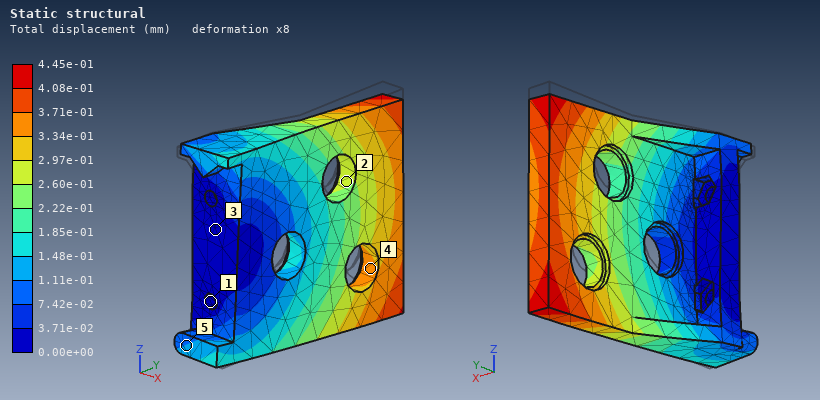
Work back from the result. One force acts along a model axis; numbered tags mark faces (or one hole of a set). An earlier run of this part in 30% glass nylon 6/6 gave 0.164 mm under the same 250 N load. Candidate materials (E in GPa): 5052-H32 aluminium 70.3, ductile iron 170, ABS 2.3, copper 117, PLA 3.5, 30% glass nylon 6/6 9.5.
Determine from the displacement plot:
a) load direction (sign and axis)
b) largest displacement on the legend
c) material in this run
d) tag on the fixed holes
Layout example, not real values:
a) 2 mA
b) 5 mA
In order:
a) -Z
b) 4.45e-01 mm
c) PLA
d) 1
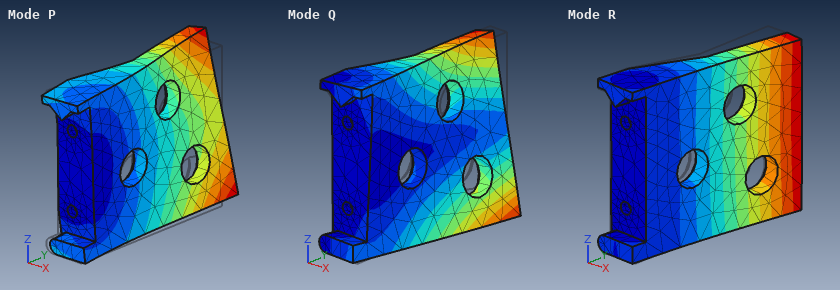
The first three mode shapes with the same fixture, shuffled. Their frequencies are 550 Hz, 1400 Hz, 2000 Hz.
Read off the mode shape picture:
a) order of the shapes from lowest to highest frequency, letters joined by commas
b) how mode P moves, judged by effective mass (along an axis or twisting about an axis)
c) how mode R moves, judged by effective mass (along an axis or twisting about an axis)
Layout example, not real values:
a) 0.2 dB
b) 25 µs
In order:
a) R, Q, P
b) along Z
c) along X
